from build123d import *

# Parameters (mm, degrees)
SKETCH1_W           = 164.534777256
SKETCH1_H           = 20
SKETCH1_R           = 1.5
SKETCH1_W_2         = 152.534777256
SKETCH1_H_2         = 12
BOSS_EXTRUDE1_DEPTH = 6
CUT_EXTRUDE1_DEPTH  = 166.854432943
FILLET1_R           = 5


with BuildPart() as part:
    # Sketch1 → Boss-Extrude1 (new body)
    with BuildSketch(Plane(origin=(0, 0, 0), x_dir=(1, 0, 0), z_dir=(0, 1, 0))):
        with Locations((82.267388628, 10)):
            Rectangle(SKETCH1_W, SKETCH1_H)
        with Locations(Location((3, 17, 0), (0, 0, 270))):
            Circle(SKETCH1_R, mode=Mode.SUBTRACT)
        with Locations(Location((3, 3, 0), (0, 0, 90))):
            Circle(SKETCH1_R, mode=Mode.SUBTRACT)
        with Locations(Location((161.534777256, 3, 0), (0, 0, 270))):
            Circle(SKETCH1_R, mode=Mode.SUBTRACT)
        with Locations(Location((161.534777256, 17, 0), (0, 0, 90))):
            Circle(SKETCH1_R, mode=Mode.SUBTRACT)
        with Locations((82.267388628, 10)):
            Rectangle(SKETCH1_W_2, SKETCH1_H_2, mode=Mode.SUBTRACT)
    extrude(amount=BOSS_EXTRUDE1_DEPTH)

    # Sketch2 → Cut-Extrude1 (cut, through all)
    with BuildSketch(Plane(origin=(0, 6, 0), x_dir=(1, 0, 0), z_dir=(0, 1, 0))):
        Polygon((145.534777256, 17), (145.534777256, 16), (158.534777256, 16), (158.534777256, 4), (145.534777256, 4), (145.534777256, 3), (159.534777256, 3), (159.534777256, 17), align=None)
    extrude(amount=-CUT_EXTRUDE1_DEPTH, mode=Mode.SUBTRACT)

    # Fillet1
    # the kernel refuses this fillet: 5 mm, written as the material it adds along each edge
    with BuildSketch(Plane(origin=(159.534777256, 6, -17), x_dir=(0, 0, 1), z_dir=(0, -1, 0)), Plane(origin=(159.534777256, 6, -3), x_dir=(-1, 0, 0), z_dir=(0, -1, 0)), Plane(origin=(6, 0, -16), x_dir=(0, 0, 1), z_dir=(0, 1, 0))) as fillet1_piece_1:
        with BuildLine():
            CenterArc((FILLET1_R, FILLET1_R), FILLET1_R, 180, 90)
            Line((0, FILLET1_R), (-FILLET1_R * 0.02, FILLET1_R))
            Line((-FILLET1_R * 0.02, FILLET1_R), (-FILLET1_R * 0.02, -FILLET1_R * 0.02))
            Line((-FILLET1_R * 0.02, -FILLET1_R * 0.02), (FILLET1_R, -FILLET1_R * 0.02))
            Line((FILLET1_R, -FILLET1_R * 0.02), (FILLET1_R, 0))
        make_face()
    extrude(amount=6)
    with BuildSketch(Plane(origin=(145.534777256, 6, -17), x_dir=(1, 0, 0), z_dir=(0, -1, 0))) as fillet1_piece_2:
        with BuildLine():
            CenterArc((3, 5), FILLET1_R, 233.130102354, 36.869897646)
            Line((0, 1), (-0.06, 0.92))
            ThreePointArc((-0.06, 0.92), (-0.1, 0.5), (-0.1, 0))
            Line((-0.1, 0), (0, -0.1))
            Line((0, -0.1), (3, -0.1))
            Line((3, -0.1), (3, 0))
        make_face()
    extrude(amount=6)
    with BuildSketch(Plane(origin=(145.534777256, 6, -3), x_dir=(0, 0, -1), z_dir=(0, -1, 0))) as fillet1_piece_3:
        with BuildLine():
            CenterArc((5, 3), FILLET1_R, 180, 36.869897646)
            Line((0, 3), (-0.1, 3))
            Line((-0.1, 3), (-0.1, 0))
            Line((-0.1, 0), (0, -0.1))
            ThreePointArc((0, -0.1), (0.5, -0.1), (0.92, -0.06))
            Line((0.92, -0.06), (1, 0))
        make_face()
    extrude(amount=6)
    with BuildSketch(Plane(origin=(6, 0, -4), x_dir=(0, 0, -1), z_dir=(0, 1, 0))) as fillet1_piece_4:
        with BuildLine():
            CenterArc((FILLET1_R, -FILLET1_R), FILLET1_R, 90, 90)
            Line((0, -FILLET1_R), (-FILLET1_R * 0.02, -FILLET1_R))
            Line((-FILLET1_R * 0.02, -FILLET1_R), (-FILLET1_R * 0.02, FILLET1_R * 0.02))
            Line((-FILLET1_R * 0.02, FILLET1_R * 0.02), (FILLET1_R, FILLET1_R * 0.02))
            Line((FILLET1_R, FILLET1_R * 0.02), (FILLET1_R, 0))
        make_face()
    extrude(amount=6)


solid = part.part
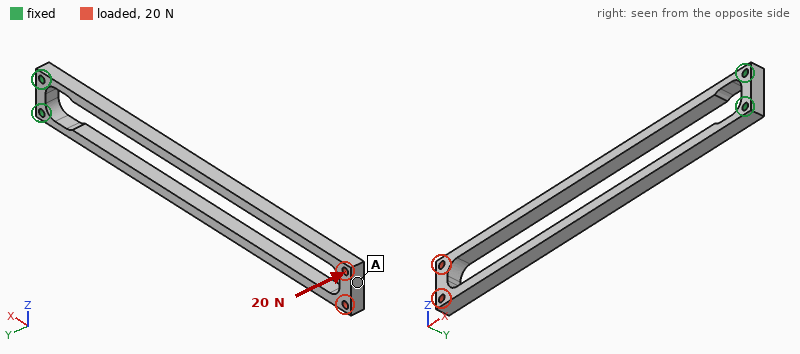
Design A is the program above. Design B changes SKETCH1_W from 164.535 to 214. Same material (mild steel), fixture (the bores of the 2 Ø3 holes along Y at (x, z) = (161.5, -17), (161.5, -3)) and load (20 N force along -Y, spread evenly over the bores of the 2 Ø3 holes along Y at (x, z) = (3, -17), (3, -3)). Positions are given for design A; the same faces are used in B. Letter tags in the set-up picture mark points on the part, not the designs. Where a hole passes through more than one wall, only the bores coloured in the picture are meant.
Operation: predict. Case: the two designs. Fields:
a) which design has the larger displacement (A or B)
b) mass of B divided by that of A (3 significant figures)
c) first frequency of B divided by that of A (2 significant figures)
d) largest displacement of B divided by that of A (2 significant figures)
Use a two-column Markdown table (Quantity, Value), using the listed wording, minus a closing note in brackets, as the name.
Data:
| Quantity | Value |
|---|---|
| which design has the larger displacement | B |
| mass of B divided by that of A | 1.70 |
| first frequency of B divided by that of A | 0.62 |
| largest displacement of B divided by that of A | 1.2 |
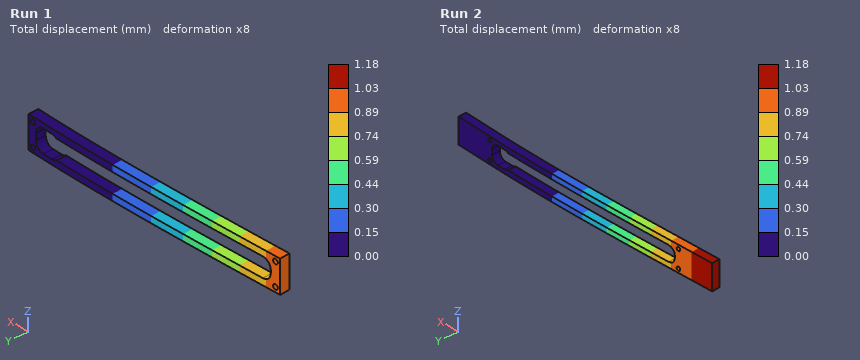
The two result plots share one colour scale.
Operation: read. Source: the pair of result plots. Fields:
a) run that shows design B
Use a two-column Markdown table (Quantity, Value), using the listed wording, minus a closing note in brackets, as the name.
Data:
| Quantity | Value |
|---|---|
| run that shows design B | Run 2 |
